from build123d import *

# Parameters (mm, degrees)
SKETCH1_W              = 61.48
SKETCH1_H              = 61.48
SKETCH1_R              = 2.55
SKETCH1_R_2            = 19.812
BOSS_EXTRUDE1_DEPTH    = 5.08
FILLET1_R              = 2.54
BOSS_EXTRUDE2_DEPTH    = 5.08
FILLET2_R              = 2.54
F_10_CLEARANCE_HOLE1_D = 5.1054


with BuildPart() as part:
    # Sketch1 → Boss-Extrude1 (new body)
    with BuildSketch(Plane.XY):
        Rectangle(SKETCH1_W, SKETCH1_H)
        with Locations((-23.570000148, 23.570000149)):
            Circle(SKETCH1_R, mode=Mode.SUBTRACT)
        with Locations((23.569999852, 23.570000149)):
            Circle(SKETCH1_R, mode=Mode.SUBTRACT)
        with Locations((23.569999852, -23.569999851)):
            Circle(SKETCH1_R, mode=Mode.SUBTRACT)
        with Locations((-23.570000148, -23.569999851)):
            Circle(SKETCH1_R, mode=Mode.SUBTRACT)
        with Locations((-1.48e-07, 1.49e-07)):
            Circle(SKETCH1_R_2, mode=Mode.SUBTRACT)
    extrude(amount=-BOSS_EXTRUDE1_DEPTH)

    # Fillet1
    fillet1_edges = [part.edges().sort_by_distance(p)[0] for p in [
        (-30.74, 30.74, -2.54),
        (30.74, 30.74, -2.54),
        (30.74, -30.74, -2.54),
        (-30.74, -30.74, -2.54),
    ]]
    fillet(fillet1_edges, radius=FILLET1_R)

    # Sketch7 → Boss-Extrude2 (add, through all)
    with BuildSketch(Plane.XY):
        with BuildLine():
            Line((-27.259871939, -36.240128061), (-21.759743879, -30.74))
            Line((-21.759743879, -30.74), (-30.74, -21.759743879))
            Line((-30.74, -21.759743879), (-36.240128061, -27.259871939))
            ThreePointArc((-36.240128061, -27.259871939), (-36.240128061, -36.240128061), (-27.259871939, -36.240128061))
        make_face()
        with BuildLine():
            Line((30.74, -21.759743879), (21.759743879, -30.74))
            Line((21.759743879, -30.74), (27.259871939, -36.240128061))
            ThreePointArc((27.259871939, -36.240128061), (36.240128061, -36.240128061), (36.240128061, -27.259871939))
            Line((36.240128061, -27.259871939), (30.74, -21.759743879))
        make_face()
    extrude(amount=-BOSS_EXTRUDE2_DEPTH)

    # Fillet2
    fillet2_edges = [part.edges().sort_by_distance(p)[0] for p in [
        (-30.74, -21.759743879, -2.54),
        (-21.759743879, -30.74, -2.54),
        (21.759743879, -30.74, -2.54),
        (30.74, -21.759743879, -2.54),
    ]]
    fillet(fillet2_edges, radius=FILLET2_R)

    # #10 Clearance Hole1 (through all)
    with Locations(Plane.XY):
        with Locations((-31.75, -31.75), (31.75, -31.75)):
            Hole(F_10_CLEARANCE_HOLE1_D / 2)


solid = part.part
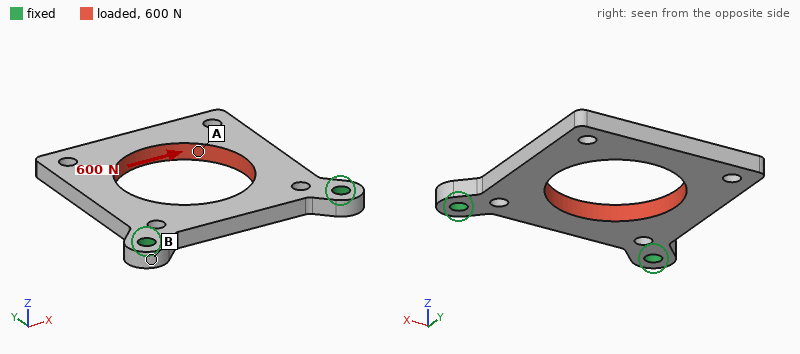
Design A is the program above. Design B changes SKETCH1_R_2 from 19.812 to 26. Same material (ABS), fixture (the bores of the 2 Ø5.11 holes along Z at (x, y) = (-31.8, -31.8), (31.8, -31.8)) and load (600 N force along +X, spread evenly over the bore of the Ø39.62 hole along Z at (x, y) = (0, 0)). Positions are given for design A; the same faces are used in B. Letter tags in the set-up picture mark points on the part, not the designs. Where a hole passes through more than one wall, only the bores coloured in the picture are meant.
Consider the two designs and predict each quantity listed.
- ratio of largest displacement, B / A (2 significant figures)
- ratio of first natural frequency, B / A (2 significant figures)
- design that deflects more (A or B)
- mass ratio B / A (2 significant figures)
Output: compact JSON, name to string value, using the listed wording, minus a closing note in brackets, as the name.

{"ratio of largest displacement, B / A": "5.0", "ratio of first natural frequency, B / A": "0.97", "design that deflects more": "B", "mass ratio B / A": "0.67"}
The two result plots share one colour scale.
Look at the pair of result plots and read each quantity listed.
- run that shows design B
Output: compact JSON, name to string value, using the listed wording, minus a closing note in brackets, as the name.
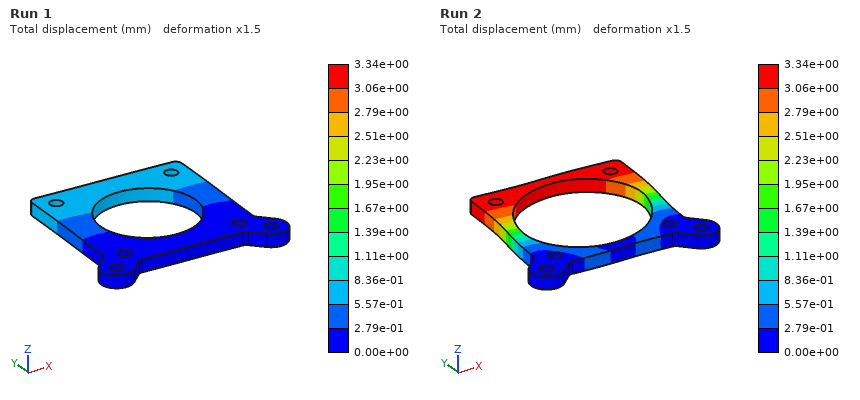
{"run that shows design B": "Run 2"}
